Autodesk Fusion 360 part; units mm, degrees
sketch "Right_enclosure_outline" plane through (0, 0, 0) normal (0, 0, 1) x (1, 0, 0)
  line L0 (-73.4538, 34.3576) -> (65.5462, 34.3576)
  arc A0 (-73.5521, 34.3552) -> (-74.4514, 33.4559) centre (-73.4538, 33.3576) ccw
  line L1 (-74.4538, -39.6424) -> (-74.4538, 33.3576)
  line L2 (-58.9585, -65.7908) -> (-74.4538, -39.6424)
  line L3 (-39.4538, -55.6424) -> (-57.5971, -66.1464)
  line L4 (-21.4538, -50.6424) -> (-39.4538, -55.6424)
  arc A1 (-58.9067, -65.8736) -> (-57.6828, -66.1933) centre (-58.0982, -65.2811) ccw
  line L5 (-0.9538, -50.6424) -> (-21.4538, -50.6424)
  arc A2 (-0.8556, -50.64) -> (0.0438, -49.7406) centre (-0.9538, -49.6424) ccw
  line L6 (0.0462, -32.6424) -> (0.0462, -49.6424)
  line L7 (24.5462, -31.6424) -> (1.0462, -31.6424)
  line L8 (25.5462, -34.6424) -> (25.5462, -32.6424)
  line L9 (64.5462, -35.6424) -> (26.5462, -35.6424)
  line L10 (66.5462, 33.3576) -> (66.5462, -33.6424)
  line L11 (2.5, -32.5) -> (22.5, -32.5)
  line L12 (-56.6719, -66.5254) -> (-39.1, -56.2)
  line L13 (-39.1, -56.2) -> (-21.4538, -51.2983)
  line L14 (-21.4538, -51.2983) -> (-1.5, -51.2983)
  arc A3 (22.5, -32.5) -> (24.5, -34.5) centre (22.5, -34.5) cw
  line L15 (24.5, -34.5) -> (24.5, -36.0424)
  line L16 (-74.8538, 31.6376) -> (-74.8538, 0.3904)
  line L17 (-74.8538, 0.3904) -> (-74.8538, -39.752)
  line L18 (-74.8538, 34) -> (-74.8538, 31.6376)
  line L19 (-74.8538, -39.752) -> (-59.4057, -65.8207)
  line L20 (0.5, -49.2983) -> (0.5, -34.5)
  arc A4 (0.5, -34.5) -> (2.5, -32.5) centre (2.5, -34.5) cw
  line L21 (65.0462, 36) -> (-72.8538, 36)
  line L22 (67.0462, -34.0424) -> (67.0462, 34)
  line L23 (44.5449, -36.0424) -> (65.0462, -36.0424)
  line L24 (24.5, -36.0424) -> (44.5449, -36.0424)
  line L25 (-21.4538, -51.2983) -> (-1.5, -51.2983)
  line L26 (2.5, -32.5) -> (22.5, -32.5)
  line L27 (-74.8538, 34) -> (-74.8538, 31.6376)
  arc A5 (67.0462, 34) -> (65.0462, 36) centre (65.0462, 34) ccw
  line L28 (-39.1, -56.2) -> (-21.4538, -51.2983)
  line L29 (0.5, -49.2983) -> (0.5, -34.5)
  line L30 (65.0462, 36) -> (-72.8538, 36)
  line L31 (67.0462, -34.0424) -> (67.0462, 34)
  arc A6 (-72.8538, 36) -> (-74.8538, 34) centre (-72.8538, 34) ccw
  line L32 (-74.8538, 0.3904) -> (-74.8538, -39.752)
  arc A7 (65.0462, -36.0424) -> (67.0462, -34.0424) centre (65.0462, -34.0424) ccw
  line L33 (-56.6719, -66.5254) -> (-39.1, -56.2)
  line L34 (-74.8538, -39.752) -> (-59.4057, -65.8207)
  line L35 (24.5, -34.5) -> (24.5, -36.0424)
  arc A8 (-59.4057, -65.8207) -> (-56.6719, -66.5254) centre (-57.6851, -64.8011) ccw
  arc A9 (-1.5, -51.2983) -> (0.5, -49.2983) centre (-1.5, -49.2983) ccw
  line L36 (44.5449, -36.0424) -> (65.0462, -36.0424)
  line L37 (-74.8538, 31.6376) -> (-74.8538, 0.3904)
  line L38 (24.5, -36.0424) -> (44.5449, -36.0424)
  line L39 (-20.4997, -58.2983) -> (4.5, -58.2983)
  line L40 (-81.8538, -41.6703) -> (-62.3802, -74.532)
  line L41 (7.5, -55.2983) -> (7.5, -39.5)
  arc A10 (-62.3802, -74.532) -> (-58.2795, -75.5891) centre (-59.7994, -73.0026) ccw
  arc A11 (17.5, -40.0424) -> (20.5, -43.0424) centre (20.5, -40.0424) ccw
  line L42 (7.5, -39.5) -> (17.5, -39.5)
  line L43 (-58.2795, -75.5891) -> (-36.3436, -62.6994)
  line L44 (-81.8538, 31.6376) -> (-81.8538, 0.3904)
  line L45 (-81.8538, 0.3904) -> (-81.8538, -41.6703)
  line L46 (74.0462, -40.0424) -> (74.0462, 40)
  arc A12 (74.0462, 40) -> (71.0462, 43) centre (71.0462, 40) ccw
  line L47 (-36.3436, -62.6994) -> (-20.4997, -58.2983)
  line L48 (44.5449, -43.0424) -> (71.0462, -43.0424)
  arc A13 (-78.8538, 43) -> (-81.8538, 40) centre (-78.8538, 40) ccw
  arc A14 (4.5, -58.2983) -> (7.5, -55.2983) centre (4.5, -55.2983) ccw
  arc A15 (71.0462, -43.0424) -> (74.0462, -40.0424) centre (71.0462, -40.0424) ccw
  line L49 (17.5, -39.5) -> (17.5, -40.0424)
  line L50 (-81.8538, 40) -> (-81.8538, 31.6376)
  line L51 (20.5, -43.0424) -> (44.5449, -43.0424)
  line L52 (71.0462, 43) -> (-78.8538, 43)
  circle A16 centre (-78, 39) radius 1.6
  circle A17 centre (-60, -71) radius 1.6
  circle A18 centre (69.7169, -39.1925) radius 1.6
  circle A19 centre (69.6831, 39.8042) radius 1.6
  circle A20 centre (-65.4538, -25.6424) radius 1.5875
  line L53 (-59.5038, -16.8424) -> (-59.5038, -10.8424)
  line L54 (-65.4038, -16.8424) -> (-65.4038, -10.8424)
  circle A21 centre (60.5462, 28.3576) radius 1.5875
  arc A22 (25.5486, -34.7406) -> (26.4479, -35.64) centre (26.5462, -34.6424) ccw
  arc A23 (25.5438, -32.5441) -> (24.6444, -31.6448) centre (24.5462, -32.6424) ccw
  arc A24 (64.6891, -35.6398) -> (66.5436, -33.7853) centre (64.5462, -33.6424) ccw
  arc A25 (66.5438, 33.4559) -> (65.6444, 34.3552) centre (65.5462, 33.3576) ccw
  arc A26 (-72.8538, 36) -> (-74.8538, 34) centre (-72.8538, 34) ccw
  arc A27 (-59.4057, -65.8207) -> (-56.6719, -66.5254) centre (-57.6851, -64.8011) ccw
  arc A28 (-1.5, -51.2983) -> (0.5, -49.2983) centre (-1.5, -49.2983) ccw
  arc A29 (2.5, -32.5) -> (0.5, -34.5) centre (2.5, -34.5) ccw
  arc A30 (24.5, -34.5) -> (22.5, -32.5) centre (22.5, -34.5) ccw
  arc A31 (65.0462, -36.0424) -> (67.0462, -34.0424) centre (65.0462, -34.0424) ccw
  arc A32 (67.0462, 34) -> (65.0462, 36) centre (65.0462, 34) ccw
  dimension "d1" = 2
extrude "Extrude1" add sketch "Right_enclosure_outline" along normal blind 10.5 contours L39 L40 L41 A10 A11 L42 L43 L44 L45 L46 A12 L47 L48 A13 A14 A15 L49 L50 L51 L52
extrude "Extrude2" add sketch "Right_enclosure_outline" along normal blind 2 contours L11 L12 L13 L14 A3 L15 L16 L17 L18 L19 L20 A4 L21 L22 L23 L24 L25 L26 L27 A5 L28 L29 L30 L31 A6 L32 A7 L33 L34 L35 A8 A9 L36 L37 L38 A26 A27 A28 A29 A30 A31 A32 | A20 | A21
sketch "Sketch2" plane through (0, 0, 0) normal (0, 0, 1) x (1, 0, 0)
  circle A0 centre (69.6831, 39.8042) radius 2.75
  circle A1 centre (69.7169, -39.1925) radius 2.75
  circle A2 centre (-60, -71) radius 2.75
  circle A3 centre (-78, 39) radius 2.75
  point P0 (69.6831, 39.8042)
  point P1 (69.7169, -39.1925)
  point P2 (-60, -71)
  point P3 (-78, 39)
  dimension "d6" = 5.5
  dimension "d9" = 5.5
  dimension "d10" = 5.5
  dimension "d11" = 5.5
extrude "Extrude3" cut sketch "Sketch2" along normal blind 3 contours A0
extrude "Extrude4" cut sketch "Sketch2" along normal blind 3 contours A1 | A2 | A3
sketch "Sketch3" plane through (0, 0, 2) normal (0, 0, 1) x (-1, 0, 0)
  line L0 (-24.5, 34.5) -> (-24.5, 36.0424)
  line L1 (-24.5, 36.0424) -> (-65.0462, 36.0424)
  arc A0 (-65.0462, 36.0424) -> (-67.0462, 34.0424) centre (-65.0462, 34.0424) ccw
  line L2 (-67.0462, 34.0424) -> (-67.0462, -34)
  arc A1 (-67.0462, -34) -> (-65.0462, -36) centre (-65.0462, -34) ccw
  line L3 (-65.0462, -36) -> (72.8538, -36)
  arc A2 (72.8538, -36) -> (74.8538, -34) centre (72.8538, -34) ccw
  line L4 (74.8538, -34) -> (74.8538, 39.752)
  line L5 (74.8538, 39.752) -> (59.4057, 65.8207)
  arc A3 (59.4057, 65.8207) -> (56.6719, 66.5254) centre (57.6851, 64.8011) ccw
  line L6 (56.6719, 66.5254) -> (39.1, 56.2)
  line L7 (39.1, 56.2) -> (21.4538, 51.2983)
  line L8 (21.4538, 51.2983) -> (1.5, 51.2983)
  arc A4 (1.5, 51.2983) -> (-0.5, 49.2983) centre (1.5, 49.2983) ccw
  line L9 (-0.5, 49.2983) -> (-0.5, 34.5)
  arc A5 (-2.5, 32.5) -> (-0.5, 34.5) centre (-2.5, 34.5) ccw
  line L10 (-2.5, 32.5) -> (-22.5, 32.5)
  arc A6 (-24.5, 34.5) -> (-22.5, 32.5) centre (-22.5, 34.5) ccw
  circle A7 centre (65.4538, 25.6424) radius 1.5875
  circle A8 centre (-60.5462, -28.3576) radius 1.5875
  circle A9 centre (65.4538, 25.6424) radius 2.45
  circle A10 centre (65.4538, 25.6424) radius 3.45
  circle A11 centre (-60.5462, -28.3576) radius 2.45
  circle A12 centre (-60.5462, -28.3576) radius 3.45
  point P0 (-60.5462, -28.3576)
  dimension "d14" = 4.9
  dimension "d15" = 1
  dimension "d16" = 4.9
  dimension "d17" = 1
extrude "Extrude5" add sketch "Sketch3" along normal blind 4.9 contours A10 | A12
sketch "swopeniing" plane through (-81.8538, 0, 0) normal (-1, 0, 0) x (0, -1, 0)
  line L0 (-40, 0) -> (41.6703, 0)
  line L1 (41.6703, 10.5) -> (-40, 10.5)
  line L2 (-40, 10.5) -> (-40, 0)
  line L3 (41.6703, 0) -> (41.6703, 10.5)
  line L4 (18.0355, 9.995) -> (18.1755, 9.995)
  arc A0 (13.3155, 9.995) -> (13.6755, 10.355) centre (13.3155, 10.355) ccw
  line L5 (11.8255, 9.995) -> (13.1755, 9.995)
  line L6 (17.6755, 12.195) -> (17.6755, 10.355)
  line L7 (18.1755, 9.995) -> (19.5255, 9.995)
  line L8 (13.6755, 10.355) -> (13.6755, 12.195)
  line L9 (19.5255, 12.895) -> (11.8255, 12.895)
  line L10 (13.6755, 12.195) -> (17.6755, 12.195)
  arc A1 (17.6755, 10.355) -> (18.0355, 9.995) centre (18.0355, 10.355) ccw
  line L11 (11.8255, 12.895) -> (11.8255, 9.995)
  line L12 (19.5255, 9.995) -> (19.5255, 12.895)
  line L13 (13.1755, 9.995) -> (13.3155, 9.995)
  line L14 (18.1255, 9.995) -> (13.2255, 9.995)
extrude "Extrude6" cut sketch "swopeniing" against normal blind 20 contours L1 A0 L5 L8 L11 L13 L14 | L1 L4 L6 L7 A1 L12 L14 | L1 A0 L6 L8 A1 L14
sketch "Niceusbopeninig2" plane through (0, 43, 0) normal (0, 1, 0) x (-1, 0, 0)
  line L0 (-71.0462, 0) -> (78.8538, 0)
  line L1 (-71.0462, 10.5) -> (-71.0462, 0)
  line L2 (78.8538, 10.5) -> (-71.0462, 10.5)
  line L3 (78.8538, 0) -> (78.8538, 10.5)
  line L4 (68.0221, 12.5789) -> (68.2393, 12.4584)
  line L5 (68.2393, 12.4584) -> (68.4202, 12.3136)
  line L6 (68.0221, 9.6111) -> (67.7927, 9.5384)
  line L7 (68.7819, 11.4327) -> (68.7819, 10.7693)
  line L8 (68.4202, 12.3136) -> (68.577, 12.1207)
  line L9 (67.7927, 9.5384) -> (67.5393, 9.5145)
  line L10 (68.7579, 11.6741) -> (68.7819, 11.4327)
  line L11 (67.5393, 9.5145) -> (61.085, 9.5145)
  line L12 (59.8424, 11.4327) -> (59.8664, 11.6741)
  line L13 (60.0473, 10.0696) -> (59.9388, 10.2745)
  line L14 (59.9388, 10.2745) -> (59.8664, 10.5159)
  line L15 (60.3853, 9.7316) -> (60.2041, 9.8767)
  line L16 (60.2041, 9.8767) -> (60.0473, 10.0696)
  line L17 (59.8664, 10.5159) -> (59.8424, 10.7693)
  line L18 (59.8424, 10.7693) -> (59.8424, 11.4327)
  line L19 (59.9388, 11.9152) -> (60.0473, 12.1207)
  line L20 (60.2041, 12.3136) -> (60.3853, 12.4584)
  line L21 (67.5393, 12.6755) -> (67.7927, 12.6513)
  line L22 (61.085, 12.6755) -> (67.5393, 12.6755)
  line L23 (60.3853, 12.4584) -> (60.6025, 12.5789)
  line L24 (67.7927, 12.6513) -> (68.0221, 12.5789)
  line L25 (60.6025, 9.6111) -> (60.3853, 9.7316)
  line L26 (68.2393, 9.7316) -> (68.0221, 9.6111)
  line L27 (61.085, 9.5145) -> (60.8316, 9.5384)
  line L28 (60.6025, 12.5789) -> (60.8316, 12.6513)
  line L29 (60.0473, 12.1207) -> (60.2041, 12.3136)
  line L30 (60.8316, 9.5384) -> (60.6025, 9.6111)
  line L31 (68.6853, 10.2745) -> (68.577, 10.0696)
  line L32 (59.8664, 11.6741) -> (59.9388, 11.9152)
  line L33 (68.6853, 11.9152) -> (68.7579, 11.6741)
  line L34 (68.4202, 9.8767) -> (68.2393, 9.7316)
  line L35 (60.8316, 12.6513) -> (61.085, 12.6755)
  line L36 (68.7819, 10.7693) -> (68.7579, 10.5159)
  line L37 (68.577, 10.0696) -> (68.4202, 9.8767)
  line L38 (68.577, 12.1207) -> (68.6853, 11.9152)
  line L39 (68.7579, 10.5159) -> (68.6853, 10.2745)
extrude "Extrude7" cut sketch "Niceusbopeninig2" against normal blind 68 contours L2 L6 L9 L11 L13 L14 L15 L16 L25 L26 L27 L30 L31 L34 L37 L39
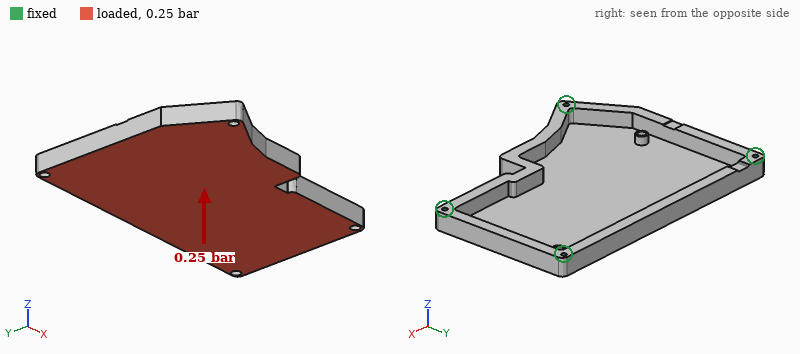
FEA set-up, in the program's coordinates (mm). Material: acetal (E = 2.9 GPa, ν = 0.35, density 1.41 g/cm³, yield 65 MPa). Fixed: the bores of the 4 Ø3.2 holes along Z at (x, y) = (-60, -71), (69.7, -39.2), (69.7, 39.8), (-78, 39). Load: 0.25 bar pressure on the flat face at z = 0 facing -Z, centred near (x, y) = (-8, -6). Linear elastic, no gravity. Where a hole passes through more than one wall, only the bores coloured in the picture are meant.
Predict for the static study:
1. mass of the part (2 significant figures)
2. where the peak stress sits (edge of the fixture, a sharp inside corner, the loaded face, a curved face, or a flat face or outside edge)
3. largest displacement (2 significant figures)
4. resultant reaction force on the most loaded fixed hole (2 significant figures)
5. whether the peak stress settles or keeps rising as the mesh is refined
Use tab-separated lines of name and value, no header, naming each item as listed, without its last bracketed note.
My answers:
mass of the part	84 g
where the peak stress sits	edge of the fixture
largest displacement	2.2 mm
resultant reaction force on the most loaded fixed hole	220 N
whether the peak stress settles or keeps rising as the mesh is refined	keeps rising
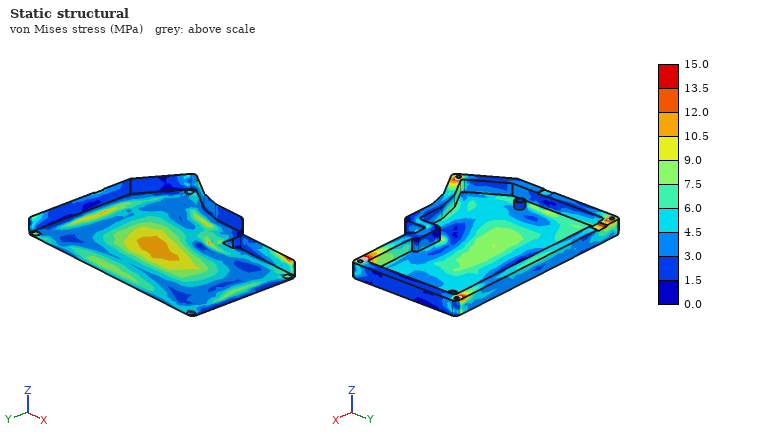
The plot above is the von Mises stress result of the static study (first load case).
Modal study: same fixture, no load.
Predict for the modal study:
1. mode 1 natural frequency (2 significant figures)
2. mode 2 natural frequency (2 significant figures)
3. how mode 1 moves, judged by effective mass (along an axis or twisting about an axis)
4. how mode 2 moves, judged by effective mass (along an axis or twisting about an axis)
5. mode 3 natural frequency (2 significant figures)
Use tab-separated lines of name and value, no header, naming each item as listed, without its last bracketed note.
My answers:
mode 1 natural frequency	380 Hz
mode 2 natural frequency	580 Hz
how mode 1 moves, judged by effective mass	along Z
how mode 2 moves, judged by effective mass	twisting about X
mode 3 natural frequency	650 Hz
